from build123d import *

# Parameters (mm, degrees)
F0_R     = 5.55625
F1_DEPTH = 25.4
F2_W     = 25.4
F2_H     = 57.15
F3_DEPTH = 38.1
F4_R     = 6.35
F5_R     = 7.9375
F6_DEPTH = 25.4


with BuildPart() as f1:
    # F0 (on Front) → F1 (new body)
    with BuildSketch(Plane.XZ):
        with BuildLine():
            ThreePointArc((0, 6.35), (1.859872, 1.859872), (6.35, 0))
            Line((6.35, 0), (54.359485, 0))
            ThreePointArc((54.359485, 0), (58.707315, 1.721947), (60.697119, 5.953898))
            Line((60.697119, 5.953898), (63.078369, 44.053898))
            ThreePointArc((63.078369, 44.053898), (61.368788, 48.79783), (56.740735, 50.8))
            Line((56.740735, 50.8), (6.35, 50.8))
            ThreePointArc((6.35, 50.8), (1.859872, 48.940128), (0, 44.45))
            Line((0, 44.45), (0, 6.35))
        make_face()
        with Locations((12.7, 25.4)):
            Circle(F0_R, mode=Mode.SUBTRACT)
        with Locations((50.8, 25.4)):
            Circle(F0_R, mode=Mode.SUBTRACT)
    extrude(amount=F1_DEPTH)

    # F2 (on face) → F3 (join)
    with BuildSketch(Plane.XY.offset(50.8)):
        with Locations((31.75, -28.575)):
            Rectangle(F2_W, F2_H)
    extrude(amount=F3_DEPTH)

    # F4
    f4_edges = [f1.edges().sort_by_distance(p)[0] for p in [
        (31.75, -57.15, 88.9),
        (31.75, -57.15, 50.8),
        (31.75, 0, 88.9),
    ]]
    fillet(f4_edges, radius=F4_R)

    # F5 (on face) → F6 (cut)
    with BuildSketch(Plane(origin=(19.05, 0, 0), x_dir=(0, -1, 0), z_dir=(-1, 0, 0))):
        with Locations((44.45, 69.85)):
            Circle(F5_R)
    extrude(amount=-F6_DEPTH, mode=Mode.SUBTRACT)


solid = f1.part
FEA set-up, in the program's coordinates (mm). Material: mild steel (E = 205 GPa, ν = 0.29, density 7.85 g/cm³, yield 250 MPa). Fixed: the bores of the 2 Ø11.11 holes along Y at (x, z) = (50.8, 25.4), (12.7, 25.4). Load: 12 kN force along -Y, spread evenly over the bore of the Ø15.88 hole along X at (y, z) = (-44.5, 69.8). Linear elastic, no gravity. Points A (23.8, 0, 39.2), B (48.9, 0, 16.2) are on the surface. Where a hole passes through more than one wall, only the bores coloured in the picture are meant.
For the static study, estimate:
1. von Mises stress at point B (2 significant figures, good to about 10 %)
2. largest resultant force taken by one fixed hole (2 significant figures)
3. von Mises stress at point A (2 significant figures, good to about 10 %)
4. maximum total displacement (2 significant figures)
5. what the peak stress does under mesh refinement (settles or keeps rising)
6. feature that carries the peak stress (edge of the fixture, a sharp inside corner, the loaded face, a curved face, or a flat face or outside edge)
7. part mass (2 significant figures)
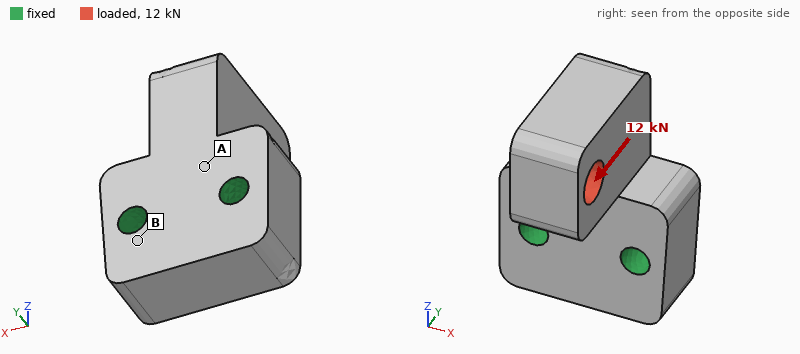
18 MPa
6.0 kN
80 MPa
77 µm
keeps rising
edge of the fixture
970 g
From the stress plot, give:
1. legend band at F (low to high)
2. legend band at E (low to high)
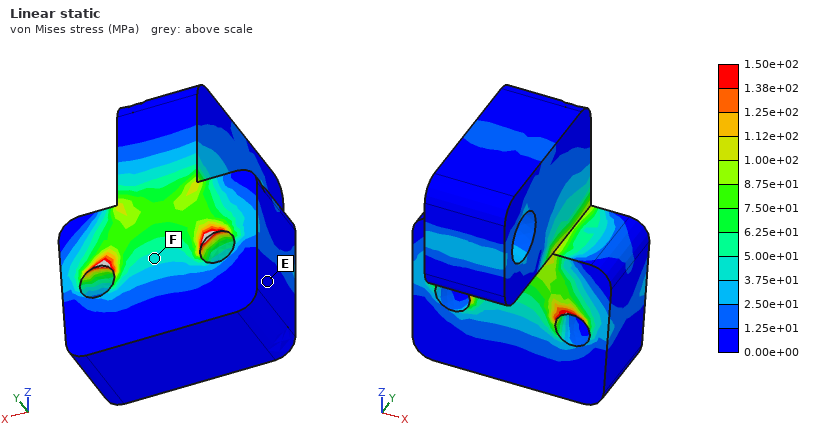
3.75e+01 to 5.00e+01 MPa
0.00e+00 to 1.25e+01 MPa
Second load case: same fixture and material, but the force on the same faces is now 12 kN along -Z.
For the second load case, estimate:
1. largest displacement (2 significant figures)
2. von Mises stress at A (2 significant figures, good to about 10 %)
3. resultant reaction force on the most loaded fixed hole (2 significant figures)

99 µm
74 MPa
6.4 kN
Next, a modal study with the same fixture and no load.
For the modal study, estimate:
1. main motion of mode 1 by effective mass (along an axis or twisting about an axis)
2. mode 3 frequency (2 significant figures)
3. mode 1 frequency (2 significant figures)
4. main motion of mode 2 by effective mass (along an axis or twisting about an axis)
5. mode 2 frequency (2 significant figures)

along Y
8100 Hz
3500 Hz
along X
5000 Hz
